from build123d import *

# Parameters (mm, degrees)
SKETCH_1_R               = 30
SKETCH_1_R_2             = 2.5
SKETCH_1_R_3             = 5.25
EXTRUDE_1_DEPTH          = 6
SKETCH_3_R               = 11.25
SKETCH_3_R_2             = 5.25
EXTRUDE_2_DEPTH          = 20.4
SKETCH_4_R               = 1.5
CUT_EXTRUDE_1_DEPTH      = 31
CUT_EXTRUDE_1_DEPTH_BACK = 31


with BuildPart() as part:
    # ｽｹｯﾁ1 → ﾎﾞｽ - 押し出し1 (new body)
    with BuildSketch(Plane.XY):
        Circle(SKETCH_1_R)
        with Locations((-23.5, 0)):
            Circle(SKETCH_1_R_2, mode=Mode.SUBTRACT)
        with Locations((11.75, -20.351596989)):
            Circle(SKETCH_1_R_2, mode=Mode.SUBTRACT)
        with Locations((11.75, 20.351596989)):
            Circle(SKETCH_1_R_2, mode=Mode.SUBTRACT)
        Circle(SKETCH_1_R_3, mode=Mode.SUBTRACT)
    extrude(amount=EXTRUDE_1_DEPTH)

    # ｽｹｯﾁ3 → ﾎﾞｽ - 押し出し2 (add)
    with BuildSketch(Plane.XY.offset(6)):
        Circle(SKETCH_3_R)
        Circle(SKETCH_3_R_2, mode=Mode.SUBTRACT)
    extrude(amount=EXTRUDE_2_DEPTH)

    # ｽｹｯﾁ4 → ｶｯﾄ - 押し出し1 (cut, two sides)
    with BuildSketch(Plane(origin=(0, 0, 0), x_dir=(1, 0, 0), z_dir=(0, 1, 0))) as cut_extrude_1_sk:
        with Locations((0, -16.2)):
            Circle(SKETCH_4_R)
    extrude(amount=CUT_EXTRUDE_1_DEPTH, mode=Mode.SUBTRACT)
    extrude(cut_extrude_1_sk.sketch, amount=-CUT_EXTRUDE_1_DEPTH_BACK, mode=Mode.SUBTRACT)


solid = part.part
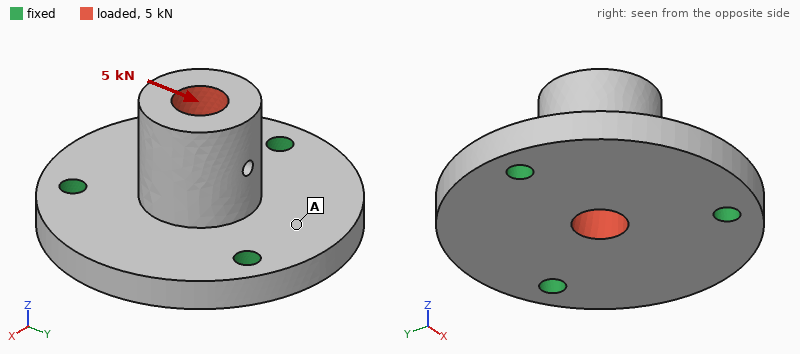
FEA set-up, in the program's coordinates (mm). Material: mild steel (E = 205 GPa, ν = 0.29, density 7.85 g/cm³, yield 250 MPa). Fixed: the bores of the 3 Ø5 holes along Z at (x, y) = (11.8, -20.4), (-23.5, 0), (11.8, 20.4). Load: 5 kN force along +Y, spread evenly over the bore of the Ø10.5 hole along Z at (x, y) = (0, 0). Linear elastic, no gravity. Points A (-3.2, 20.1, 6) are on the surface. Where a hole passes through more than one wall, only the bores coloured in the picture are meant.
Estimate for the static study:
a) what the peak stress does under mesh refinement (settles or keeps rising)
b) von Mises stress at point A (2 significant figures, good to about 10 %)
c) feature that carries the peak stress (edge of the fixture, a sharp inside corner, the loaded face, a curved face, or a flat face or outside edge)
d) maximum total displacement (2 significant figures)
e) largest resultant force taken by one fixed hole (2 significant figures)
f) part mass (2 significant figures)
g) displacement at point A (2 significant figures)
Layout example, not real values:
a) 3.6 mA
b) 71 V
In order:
a) keeps rising
b) 17 MPa
c) edge of the fixture
d) 19 µm
e) 2.3 kN
f) 180 g
g) 4.8 µm
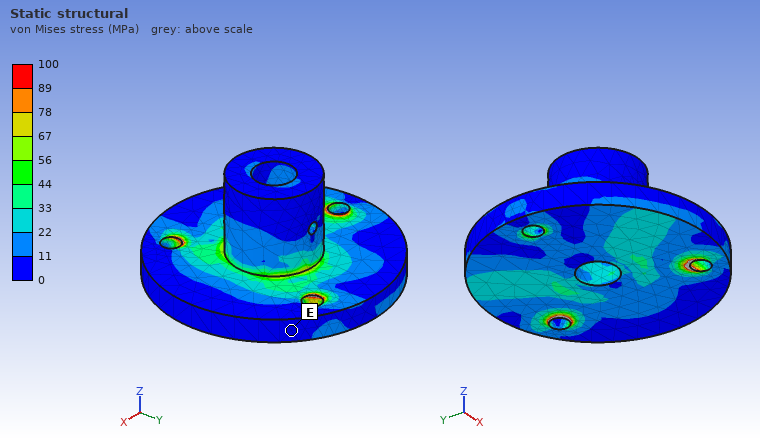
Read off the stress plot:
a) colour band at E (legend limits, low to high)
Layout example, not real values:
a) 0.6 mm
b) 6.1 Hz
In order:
a) 0 to 11 MPa
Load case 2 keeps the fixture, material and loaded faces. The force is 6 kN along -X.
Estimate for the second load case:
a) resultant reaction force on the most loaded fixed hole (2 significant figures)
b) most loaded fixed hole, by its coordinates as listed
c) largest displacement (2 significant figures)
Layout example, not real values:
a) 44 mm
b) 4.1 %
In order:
a) 3.0 kN
b) (-23.5, 0)
c) 23 µm
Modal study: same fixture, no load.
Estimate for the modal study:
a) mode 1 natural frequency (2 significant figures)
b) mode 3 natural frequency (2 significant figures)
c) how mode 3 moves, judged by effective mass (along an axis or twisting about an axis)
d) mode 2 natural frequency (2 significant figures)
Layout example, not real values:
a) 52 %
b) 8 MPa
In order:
a) 10 kHz
b) 12 kHz
c) along Z
d) 10 kHz
